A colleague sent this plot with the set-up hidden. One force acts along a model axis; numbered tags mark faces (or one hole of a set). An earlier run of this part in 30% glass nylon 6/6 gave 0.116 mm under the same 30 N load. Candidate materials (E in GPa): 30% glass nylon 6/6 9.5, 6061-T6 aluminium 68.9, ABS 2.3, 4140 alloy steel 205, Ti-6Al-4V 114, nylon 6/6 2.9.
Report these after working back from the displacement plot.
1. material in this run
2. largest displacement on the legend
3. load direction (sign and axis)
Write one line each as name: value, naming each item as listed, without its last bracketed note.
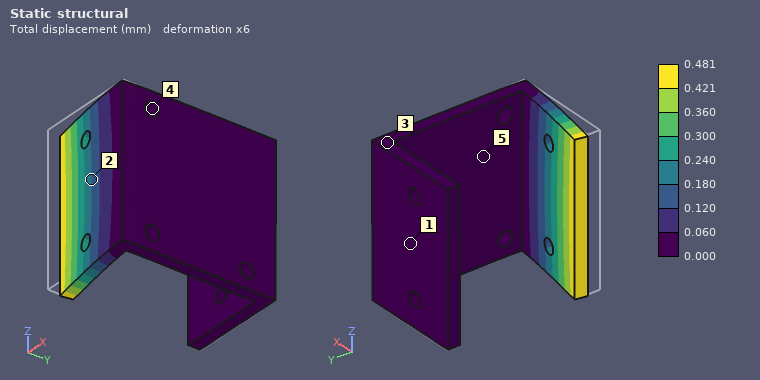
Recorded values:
material in this run: ABS
largest displacement on the legend: 0.481 mm
load direction: +Y
